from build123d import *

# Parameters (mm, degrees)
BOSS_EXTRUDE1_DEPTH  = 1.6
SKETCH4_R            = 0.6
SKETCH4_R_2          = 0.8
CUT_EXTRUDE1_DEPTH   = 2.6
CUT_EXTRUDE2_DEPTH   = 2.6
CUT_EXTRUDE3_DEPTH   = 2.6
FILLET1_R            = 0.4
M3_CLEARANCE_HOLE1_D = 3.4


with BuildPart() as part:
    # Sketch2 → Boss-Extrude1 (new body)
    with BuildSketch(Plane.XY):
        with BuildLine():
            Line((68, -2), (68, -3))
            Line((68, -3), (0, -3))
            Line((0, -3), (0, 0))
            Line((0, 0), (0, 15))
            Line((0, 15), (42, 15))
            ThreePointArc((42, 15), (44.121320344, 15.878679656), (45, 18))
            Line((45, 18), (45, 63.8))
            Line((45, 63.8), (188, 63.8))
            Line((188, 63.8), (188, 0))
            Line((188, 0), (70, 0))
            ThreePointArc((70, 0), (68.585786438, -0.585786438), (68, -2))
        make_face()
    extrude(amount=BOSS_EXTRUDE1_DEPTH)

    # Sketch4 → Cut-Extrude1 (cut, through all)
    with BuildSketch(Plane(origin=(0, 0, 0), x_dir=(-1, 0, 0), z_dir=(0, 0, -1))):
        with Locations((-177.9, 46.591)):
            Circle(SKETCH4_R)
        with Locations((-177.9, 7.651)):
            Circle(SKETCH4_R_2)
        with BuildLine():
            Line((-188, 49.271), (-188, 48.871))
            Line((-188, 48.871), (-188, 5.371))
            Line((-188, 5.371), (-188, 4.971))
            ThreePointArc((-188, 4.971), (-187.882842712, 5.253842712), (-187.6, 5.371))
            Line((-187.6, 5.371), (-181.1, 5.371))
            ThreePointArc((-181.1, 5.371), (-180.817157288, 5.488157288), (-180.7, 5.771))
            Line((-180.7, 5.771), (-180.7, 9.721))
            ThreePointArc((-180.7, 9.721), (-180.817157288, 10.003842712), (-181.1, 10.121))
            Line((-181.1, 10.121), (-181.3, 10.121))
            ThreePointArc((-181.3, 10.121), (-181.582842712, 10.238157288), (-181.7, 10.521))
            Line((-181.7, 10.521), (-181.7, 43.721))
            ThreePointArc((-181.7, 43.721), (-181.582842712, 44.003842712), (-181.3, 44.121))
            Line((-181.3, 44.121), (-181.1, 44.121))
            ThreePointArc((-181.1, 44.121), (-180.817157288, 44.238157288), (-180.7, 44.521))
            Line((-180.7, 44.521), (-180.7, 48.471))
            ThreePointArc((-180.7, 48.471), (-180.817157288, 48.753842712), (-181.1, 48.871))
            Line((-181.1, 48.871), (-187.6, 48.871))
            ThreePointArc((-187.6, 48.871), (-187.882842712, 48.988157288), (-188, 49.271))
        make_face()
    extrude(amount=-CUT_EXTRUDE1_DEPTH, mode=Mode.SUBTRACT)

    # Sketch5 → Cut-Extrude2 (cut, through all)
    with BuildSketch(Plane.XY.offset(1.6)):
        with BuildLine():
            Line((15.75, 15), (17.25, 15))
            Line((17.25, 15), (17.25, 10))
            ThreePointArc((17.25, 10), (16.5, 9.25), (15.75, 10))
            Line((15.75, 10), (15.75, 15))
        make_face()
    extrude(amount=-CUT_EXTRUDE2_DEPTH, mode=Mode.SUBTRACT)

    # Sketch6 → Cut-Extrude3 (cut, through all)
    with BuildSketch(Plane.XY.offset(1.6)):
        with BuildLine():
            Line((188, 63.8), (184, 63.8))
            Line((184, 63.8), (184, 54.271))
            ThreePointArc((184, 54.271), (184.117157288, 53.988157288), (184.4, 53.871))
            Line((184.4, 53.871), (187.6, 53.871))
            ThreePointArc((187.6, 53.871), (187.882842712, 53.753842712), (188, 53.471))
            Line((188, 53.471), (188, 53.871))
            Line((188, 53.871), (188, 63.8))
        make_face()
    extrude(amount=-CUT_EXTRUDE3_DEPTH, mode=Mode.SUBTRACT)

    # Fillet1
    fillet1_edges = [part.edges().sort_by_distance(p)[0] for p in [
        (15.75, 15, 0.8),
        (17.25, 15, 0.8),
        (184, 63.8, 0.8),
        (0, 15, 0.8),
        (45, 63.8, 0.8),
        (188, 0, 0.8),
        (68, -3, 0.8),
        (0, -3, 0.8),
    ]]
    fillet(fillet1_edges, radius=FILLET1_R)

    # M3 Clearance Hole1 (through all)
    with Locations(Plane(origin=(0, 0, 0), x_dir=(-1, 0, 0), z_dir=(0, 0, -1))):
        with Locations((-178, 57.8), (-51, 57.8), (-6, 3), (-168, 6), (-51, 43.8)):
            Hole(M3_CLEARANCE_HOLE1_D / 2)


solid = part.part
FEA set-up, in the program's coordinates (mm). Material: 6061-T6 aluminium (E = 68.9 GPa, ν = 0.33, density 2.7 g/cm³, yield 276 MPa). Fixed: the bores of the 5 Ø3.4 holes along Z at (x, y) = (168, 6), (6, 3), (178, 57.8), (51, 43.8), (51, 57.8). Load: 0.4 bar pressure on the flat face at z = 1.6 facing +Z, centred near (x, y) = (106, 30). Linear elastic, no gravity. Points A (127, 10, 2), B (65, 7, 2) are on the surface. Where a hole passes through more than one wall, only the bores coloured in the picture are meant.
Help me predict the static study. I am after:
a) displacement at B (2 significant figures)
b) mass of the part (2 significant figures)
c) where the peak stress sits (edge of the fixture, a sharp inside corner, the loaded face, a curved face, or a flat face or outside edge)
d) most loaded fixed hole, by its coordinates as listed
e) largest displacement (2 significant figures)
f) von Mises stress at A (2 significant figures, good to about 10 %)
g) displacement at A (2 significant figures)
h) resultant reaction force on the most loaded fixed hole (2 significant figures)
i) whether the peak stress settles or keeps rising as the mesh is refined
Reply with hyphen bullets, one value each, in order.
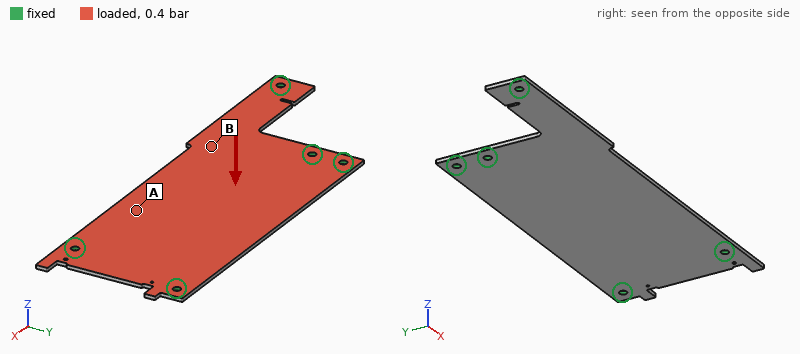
- 1.0 mm
- 42 g
- edge of the fixture
- (51, 43.8)
- 1.7 mm
- 56 MPa
- 1.1 mm
- 170 N
- keeps rising
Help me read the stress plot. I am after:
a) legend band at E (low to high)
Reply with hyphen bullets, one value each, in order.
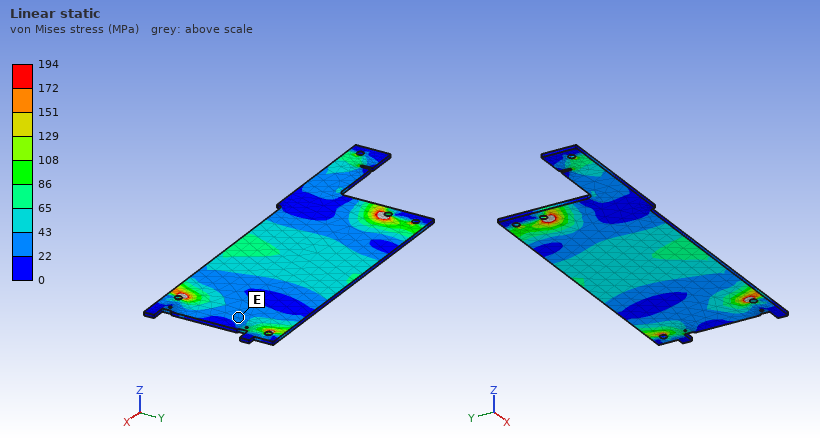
- 22 to 43 MPa
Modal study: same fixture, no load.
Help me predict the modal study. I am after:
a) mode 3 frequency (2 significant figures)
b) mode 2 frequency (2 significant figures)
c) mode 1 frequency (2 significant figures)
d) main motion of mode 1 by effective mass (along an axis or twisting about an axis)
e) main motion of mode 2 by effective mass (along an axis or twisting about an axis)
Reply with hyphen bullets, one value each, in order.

- 1200 Hz
- 700 Hz
- 480 Hz
- along Z
- twisting about X
